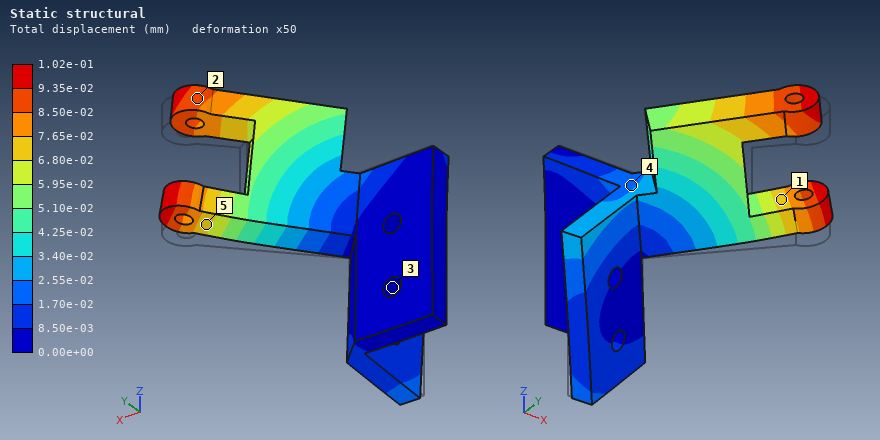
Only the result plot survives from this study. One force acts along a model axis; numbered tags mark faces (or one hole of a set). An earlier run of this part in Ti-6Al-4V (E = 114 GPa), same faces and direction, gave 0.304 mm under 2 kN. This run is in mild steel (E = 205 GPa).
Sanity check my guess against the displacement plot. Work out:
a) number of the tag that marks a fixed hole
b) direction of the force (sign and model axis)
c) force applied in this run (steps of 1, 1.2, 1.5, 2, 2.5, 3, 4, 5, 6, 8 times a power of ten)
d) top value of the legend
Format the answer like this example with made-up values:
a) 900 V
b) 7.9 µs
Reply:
a) 3
b) +Z
c) 1.2 kN
d) 1.02e-01 mm
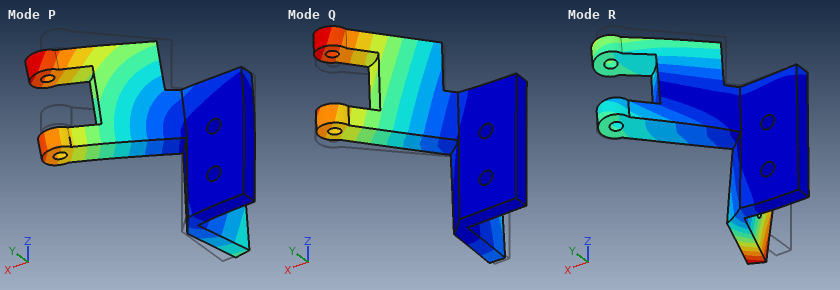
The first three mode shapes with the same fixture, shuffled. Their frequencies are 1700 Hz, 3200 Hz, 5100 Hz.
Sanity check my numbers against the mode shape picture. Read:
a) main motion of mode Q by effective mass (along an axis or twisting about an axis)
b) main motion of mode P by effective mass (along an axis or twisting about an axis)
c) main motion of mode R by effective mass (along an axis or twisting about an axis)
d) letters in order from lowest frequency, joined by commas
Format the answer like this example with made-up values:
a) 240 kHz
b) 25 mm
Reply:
a) along Y
b) along Z
c) along X
d) Q, P, R
